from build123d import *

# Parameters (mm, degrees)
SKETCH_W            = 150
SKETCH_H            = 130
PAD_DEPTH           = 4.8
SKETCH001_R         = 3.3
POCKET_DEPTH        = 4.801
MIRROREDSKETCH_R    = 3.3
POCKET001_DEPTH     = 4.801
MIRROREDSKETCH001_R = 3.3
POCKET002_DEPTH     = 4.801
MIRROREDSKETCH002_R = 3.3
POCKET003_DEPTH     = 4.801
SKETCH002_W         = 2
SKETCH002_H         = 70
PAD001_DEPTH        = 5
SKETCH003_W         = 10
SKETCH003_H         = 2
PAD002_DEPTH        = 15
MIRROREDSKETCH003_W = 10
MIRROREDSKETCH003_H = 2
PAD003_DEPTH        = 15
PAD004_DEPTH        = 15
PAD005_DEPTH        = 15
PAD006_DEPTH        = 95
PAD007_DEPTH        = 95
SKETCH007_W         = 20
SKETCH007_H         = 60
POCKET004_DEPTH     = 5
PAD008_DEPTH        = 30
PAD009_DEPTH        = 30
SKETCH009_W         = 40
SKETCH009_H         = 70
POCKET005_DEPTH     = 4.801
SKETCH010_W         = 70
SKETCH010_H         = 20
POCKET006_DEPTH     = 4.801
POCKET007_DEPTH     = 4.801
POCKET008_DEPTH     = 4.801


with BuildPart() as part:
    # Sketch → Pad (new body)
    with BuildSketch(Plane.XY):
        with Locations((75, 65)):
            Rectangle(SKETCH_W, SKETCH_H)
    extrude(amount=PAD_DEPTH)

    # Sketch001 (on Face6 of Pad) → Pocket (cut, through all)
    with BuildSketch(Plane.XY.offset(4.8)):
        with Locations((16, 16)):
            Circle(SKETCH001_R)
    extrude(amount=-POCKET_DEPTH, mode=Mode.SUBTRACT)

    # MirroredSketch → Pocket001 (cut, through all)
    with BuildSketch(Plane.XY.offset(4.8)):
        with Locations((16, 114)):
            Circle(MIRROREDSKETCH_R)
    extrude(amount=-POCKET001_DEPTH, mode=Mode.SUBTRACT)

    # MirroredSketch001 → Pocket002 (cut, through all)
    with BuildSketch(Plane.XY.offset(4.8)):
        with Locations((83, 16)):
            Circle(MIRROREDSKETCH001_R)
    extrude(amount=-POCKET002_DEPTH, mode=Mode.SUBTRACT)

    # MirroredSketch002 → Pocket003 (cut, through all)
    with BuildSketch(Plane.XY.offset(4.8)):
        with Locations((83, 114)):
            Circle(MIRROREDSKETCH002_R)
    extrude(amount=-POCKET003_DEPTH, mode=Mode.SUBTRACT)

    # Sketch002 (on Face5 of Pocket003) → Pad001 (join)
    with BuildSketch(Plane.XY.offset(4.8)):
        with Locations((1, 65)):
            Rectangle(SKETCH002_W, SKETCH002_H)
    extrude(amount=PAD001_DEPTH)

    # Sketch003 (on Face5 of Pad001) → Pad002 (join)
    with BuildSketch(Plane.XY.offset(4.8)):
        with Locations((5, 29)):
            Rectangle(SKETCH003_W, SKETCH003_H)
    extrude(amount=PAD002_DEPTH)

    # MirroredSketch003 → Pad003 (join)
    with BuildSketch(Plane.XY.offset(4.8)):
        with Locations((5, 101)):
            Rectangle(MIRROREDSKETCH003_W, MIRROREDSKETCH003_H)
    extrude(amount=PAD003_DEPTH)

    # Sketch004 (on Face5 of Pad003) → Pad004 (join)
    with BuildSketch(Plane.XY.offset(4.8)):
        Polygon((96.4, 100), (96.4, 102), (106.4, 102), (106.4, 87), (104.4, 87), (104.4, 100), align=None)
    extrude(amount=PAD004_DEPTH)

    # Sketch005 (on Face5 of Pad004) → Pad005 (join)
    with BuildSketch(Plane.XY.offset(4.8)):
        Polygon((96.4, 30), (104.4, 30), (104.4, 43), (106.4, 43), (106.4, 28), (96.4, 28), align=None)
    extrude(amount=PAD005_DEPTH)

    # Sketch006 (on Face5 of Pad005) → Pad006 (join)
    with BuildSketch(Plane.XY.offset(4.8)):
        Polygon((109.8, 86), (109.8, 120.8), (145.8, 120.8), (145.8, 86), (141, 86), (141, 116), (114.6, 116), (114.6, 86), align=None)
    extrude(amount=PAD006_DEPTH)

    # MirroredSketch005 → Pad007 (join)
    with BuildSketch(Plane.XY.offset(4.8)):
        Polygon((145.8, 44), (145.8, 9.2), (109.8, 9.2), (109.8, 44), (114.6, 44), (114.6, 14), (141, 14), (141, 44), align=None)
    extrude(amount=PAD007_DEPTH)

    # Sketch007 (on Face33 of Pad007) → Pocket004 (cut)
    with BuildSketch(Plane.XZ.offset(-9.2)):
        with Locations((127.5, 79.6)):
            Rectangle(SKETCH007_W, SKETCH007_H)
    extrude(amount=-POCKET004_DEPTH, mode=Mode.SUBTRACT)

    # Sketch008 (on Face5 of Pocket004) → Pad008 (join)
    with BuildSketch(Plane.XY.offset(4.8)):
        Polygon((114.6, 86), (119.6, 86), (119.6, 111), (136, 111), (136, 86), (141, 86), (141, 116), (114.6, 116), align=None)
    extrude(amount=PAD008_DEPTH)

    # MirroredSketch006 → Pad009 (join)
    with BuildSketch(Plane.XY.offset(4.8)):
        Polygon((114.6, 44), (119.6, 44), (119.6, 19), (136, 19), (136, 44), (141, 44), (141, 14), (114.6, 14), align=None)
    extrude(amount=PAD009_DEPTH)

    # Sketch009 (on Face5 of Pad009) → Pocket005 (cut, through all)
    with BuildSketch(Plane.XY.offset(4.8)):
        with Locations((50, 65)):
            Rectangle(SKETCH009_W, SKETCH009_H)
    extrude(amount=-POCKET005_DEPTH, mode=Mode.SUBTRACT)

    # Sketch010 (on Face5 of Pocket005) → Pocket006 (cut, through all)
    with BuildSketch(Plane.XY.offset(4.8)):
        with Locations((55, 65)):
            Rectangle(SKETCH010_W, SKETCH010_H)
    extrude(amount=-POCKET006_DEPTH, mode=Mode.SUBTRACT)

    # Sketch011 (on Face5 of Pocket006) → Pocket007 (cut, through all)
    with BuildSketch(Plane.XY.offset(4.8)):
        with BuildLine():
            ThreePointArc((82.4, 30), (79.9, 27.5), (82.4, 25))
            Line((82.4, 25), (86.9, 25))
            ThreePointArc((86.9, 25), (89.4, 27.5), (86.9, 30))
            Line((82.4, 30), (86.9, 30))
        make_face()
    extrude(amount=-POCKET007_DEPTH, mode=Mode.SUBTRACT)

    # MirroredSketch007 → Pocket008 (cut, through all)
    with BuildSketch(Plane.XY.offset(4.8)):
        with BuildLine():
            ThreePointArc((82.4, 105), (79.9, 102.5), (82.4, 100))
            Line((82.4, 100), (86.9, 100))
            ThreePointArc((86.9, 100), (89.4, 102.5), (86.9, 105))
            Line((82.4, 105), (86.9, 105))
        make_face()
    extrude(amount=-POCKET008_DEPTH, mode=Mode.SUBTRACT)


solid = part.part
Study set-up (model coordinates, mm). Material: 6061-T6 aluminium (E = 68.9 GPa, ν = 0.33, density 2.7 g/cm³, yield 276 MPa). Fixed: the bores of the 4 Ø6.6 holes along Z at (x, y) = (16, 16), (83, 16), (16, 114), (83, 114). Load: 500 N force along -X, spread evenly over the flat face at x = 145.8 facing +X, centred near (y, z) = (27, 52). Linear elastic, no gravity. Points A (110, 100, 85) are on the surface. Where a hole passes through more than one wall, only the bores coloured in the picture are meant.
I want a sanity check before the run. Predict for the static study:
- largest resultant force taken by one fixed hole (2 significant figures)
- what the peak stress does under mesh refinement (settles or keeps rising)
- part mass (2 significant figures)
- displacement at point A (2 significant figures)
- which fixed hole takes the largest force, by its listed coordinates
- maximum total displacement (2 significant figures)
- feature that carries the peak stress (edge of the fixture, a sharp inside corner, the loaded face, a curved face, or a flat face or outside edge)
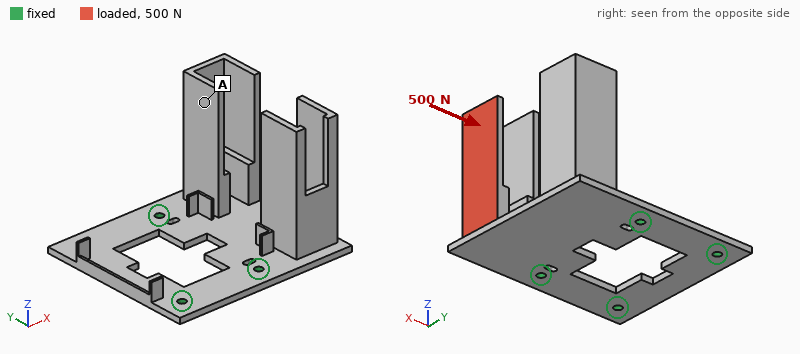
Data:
420 N
keeps rising
500 g
0.77 mm
(83, 16)
1.9 mm
edge of the fixture
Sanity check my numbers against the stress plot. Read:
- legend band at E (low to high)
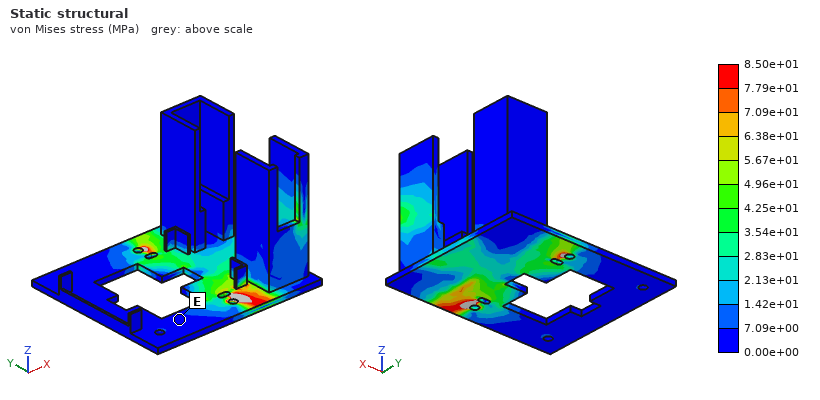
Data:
0.00e+00 to 7.09e+00 MPa
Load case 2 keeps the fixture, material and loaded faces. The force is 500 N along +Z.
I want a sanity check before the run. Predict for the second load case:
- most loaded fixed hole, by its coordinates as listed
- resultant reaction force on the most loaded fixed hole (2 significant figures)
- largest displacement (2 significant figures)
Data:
(83, 16)
460 N
1.6 mm
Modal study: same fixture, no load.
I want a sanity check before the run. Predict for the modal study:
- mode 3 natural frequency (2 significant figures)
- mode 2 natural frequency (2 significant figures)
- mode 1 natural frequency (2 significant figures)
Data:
470 Hz
410 Hz
210 Hz
